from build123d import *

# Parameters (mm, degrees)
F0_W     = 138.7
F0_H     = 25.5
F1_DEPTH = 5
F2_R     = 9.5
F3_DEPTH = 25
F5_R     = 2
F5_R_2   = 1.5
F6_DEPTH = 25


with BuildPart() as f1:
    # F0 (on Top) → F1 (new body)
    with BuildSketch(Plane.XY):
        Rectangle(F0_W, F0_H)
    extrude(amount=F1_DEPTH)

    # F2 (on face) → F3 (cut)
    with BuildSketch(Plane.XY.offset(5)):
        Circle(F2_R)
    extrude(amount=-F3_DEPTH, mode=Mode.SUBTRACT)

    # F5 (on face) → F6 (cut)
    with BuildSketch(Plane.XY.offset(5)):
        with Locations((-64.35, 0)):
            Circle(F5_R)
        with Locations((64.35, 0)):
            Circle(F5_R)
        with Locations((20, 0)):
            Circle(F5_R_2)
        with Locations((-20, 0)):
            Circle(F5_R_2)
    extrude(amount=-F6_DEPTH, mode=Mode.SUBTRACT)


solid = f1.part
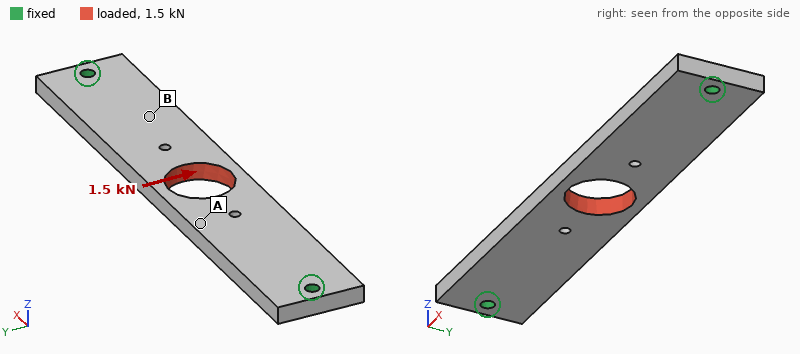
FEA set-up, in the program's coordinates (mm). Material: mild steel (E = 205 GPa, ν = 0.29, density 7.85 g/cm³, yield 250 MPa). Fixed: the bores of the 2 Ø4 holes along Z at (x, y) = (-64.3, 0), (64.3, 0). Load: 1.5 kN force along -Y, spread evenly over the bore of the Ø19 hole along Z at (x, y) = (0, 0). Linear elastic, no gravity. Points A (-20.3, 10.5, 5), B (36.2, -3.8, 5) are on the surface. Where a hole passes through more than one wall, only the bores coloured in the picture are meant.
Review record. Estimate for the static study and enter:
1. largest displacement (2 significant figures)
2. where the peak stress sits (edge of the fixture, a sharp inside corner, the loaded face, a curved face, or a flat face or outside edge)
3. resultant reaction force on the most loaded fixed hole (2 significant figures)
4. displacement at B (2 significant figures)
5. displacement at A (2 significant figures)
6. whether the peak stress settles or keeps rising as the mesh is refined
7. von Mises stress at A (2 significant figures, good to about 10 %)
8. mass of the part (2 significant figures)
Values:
38 µm
edge of the fixture
750 N
21 µm
32 µm
keeps rising
32 MPa
130 g
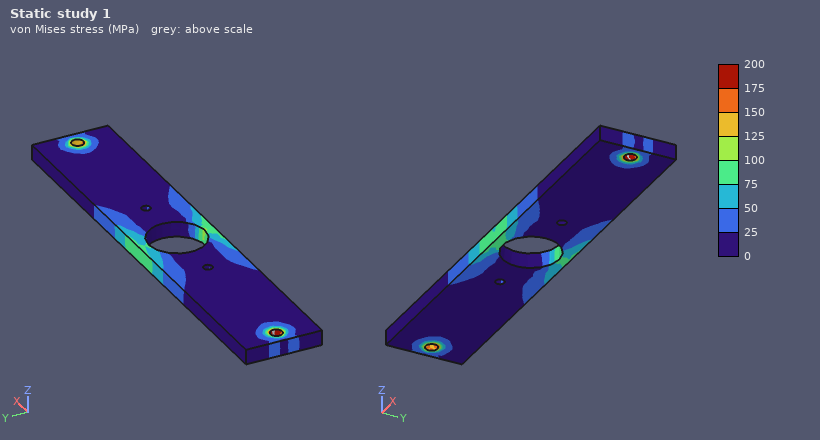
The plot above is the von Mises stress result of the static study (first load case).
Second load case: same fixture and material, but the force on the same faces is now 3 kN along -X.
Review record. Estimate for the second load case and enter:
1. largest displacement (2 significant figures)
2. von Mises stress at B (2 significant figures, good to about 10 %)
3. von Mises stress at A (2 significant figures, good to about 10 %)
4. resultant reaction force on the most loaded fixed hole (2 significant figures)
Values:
4.4 µm
12 MPa
12 MPa
1.5 kN
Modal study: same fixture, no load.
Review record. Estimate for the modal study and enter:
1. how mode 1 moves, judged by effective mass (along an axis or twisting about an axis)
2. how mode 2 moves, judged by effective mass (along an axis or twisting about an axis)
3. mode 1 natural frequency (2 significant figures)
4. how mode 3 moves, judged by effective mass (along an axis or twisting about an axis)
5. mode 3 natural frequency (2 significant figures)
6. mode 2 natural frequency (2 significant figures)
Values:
along Z
twisting about Y
1500 Hz
along Y
4400 Hz
4000 Hz
